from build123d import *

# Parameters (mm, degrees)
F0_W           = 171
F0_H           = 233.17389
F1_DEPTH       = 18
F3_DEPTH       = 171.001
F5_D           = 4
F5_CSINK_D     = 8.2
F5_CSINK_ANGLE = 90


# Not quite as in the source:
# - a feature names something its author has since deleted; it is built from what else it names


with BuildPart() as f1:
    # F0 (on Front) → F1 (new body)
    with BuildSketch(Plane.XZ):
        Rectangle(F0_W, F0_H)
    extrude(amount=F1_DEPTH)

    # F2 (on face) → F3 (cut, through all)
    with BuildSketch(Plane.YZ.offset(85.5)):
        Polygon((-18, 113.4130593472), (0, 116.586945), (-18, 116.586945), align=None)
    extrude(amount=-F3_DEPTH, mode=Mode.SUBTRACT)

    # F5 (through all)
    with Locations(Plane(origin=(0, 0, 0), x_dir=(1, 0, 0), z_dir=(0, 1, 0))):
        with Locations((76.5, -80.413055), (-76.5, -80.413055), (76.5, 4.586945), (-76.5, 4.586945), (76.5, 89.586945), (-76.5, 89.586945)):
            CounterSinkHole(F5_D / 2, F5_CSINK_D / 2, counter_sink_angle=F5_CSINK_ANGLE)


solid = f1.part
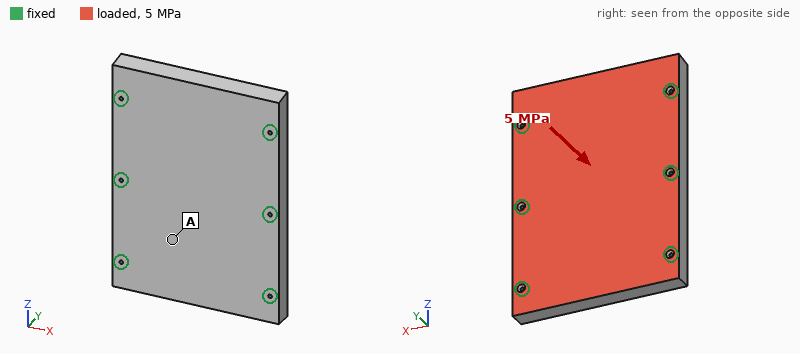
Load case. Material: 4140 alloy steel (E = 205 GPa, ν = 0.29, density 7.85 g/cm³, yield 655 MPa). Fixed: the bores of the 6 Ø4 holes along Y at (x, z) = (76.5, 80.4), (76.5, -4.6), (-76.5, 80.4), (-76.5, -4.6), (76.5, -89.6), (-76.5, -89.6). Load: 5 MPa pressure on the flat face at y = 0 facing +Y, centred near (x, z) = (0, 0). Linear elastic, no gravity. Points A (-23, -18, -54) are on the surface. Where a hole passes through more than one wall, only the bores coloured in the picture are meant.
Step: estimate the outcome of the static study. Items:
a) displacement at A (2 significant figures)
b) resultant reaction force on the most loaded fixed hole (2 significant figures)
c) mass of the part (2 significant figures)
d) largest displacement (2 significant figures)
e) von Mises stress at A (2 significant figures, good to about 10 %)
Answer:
0.15 mm
35 kN
5.6 kg
0.21 mm
100 MPa
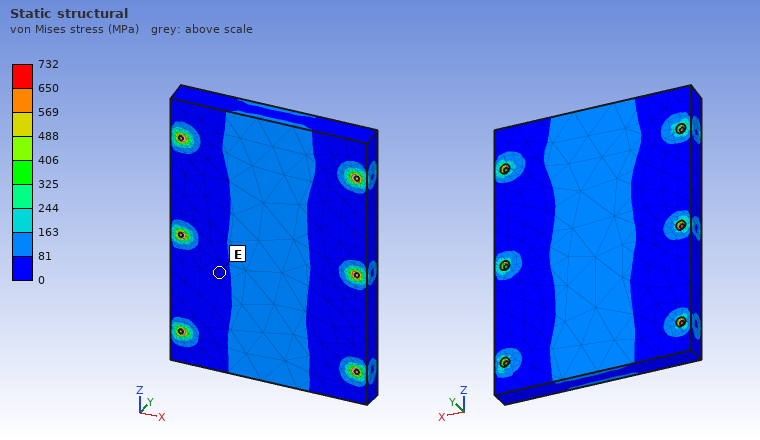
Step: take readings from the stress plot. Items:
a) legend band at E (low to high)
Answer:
0 to 81 MPa
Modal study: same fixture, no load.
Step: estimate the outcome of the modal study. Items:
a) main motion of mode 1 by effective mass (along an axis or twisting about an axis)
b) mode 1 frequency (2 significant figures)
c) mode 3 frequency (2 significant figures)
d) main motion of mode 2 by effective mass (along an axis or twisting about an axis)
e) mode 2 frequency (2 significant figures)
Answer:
along Y
2500 Hz
4000 Hz
twisting about X
2900 Hz
